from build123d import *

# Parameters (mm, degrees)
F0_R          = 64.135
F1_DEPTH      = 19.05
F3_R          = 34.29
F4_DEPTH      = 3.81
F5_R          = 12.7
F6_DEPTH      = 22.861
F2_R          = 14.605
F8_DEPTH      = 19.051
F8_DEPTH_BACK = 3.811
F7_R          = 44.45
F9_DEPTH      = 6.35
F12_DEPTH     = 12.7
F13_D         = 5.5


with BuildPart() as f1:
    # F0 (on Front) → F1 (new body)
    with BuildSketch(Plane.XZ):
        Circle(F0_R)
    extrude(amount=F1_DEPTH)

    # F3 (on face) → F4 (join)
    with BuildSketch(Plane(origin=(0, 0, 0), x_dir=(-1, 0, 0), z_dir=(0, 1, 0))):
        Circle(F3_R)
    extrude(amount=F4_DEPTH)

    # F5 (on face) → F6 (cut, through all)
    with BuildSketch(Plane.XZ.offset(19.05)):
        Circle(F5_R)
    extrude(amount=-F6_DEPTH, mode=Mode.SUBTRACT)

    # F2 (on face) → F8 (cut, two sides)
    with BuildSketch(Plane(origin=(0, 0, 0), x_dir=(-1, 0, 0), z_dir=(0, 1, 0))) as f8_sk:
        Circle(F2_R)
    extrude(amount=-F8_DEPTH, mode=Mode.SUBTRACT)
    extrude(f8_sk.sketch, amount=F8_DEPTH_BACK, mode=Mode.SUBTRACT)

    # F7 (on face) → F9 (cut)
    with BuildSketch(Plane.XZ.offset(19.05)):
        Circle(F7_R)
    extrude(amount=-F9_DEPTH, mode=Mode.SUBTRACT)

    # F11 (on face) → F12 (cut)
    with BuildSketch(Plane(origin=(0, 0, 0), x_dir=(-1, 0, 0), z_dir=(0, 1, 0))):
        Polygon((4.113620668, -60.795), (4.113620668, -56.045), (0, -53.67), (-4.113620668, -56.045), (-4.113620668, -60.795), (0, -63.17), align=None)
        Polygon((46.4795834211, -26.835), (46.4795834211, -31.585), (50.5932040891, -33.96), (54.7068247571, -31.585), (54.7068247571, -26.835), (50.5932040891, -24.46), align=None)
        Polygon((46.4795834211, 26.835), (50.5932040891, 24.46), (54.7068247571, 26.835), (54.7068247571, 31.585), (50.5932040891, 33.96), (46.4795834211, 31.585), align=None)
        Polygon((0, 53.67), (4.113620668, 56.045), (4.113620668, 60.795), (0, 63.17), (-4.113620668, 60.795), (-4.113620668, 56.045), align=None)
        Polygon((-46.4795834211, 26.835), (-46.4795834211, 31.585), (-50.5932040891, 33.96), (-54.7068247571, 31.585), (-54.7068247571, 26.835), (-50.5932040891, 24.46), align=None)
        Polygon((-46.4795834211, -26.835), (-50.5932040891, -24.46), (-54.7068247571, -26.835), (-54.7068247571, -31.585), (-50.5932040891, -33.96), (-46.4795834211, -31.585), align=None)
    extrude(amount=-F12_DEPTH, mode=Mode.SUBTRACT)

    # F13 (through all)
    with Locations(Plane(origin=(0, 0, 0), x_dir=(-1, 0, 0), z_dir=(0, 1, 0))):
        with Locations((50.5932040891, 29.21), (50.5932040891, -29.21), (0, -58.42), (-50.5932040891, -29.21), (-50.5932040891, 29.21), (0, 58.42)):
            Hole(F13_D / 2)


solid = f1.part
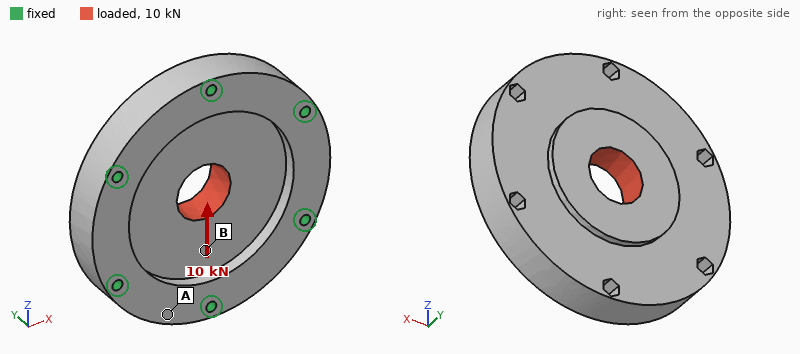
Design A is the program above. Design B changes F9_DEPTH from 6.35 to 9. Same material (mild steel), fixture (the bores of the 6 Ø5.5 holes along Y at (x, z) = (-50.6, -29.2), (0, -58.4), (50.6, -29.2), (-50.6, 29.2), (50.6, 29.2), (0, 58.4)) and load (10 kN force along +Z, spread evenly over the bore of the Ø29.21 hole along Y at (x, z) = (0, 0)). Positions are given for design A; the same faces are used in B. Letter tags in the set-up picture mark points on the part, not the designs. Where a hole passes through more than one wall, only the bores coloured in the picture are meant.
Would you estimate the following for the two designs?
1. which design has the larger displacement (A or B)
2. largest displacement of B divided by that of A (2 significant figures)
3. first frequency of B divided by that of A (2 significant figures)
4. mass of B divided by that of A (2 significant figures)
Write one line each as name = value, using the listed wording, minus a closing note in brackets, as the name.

which design has the larger displacement = B
largest displacement of B divided by that of A = 1.2
first frequency of B divided by that of A = 1.0
mass of B divided by that of A = 0.93
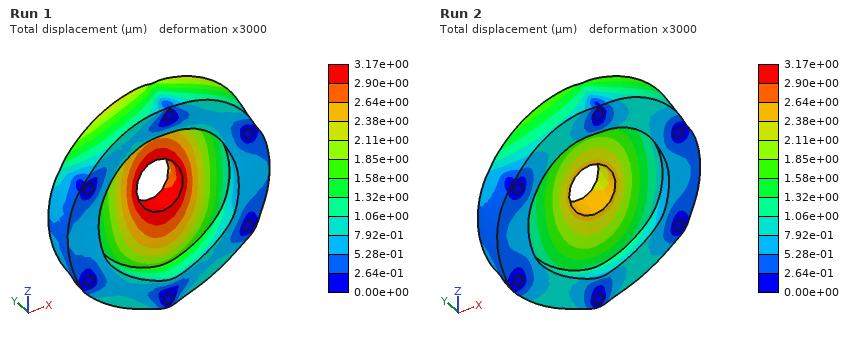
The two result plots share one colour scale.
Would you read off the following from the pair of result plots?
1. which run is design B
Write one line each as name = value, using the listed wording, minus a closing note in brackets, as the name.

which run is design B = Run 1
